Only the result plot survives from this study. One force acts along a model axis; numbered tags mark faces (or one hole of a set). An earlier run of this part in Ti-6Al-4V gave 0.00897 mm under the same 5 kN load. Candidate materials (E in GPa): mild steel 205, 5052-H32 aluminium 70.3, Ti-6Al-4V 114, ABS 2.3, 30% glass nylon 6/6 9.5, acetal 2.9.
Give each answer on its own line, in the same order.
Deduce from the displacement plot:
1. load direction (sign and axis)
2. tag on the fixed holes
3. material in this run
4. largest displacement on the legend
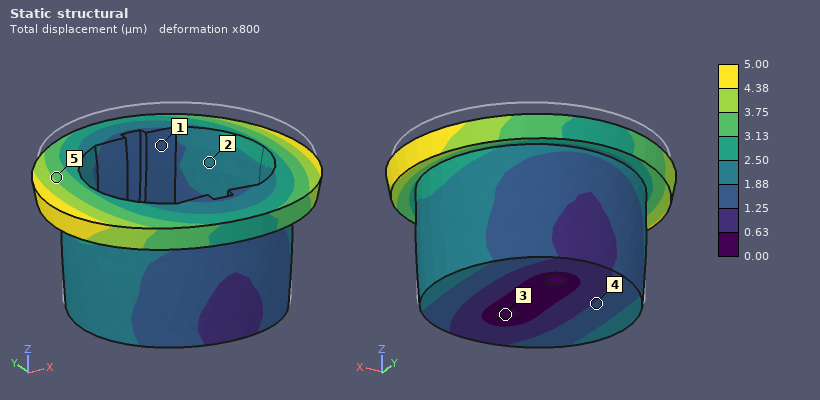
-Z
3
mild steel
5.00 µm
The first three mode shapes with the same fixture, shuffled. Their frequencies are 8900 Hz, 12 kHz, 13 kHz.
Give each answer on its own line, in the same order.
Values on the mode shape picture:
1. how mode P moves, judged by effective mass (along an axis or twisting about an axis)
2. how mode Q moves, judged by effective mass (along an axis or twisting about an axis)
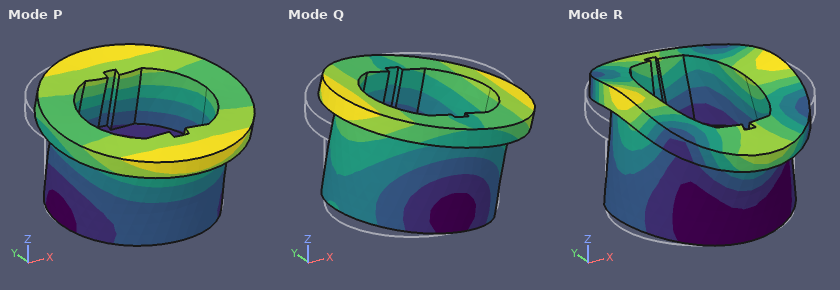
along Y
along X
